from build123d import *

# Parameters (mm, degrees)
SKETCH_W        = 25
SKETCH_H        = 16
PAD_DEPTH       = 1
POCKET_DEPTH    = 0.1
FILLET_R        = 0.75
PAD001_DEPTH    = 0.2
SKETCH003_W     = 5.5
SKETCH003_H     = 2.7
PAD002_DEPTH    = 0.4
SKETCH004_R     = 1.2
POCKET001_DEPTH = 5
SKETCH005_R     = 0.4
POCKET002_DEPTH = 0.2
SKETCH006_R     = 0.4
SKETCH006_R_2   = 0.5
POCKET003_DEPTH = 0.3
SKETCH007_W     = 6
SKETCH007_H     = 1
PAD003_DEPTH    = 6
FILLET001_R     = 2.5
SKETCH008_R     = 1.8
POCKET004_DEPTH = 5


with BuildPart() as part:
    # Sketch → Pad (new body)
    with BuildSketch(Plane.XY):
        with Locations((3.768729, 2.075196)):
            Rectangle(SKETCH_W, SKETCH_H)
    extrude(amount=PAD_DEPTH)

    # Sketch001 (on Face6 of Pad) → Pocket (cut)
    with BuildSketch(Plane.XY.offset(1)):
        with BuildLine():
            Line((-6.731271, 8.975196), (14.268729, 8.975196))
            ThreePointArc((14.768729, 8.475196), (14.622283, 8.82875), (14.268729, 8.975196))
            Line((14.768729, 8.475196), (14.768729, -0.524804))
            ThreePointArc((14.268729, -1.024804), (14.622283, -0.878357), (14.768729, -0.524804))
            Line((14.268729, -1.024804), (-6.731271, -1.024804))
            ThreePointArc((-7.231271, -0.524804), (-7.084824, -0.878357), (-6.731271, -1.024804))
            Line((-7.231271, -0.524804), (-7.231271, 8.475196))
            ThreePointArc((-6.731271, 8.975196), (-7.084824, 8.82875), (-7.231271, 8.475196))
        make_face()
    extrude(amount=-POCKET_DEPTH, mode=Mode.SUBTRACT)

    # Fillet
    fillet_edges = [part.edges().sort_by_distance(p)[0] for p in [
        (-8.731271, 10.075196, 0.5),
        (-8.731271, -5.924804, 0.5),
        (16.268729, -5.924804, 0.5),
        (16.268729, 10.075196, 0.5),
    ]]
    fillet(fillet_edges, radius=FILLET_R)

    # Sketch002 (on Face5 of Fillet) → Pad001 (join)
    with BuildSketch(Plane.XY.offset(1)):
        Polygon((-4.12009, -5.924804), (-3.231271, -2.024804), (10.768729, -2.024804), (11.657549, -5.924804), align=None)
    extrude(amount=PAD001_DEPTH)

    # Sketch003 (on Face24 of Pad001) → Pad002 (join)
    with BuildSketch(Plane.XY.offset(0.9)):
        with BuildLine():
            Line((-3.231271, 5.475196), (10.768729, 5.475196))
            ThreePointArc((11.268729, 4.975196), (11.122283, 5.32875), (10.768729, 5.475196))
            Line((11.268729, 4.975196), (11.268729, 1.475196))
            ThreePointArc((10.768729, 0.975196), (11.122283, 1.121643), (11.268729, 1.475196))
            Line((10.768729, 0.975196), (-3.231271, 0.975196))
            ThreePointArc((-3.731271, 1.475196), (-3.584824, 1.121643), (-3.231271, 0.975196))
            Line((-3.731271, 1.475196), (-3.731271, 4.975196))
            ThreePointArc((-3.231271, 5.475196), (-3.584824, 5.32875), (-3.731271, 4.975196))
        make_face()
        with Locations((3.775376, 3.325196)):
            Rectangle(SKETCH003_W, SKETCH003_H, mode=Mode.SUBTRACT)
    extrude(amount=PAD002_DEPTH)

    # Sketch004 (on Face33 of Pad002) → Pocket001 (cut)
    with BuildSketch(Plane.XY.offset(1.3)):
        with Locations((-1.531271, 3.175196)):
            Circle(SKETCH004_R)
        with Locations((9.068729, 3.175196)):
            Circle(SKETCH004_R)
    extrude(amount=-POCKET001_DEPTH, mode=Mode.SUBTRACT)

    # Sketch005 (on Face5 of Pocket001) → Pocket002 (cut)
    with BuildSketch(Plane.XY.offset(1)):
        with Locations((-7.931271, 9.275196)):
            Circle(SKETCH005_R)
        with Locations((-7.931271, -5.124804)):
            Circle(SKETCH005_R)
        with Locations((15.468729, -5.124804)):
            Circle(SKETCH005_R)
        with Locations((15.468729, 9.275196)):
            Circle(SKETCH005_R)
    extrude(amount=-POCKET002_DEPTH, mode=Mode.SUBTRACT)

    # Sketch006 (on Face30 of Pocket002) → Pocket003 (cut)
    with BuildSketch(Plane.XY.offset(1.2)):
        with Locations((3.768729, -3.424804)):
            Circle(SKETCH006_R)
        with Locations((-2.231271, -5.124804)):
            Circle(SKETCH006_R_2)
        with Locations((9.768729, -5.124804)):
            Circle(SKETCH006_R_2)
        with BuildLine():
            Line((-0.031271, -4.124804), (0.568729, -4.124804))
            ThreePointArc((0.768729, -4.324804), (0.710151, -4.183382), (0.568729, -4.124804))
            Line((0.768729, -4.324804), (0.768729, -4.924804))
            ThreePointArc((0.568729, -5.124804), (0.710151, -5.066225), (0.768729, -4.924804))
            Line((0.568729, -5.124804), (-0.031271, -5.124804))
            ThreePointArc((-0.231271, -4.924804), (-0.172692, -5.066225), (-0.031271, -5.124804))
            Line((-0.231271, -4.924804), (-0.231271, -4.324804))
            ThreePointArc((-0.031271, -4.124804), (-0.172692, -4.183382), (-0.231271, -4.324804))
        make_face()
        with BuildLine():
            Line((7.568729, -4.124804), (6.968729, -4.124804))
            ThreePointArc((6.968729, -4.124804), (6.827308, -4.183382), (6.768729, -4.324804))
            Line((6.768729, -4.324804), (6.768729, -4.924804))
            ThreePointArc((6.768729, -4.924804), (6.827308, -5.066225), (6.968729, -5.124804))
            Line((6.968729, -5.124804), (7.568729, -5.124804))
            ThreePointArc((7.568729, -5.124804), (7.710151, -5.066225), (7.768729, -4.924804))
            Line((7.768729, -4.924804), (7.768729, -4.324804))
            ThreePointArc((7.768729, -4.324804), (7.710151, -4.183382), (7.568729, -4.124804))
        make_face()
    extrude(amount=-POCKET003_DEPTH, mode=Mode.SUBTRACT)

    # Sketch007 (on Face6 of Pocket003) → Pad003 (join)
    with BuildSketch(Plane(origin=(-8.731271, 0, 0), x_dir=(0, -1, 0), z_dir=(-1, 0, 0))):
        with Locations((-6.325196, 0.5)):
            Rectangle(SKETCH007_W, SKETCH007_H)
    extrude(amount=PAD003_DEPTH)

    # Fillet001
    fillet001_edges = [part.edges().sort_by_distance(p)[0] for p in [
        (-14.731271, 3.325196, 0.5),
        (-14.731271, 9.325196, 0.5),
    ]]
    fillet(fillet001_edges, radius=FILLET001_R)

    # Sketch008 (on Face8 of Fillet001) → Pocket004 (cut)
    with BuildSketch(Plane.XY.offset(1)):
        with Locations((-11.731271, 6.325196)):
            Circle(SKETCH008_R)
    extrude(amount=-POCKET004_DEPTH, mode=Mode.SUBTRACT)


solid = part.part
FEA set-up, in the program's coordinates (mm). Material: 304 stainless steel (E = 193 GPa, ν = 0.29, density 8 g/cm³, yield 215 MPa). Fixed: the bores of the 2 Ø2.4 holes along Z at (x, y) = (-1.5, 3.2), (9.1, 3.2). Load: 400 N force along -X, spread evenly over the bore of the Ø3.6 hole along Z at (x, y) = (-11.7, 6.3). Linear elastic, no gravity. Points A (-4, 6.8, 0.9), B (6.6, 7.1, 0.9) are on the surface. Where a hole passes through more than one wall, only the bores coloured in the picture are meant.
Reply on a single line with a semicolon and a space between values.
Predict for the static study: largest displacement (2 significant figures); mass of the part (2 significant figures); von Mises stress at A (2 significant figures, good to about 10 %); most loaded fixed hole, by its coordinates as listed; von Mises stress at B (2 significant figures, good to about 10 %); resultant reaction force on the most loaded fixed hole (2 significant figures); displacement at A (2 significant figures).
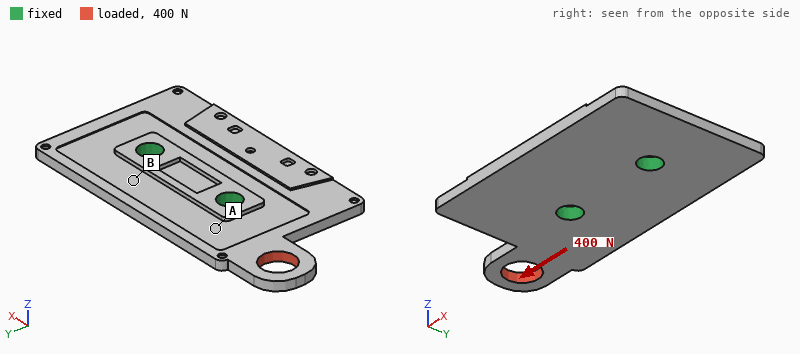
9.9 µm; 3.4 g; 60 MPa; (-1.5, 3.2); 21 MPa; 330 N; 2.0 µm
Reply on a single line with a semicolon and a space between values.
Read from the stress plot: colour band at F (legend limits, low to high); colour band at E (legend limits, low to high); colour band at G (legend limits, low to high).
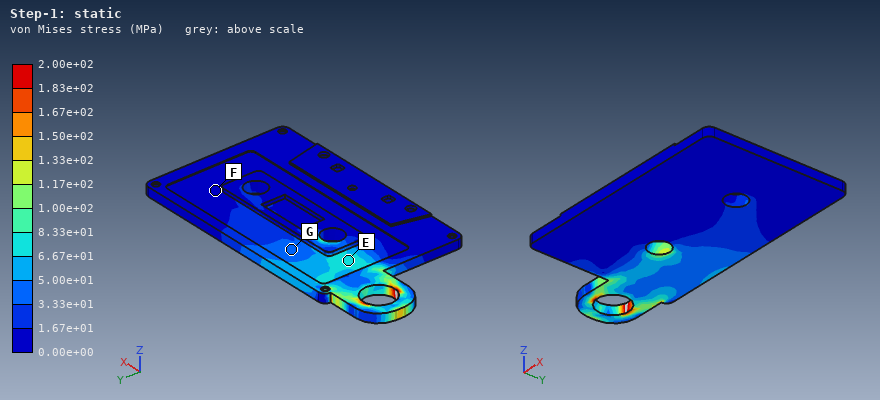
0.00e+00 to 1.67e+01 MPa; 6.67e+01 to 8.33e+01 MPa; 3.33e+01 to 5.00e+01 MPa
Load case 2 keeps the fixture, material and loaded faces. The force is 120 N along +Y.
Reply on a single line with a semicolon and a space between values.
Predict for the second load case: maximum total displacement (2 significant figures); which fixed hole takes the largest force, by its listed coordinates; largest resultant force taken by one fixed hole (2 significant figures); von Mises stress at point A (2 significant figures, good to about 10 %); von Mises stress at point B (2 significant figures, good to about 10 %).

13 µm; (-1.5, 3.2); 200 N; 17 MPa; 14 MPa
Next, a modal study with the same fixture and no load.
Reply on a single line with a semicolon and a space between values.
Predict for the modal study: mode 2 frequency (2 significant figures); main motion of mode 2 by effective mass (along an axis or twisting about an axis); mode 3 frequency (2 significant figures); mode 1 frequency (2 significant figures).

9800 Hz; along Z; 12 kHz; 7200 Hz
